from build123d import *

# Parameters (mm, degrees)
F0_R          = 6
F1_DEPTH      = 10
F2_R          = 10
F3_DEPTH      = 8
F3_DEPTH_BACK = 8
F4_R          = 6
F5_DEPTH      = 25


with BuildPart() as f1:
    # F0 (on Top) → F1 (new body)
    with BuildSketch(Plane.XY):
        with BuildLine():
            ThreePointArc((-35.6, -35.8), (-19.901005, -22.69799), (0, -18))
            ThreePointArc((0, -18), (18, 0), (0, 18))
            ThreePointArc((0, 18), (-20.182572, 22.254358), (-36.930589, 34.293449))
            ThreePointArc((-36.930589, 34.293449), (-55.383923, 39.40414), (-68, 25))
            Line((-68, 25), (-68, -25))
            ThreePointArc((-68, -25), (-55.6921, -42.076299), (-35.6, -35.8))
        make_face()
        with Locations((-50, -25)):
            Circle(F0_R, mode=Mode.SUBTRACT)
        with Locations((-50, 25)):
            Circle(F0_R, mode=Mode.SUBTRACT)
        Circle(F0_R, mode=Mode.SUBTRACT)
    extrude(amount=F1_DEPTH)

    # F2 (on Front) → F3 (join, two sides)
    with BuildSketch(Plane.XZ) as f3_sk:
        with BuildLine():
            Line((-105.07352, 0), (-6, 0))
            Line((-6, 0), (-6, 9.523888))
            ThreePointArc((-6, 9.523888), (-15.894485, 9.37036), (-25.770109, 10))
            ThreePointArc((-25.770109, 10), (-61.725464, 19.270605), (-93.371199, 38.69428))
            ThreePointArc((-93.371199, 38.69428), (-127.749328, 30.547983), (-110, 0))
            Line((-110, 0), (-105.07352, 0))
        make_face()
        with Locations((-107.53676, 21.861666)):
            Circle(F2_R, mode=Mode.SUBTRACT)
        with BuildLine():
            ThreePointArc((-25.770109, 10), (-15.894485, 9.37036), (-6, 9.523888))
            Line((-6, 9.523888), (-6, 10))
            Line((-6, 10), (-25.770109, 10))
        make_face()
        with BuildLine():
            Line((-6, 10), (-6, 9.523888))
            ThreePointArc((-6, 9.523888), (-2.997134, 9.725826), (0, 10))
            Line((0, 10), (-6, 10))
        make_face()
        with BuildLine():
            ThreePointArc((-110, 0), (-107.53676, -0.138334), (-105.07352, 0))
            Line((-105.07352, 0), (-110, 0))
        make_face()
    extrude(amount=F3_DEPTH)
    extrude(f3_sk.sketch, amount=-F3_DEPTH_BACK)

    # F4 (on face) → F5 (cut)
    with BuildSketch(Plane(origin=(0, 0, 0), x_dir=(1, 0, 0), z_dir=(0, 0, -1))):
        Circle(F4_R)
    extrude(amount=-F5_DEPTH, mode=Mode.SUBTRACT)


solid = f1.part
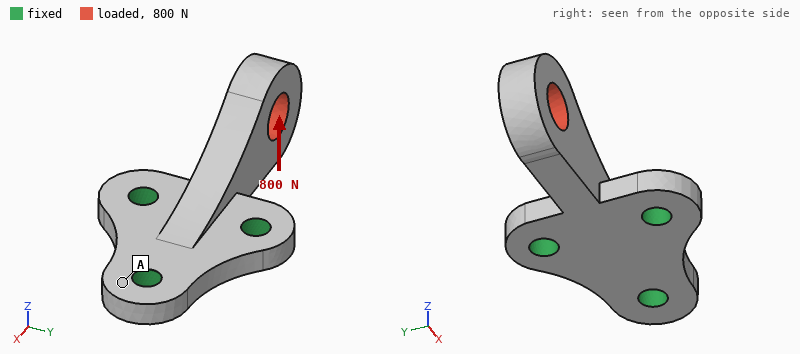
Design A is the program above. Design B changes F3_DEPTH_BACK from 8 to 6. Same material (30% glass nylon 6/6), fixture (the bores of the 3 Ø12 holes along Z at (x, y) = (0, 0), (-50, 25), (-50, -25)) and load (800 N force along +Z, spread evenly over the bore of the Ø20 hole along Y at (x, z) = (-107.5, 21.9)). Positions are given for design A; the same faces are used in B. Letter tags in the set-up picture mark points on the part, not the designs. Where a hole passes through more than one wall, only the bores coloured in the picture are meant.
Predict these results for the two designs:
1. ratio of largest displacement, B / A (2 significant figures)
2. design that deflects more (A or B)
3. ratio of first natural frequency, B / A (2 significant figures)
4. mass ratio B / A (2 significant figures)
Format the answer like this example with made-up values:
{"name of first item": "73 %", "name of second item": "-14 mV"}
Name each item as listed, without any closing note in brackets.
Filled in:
{"ratio of largest displacement, B / A": "1.1", "design that deflects more": "B", "ratio of first natural frequency, B / A": "1.0", "mass ratio B / A": "0.95"}
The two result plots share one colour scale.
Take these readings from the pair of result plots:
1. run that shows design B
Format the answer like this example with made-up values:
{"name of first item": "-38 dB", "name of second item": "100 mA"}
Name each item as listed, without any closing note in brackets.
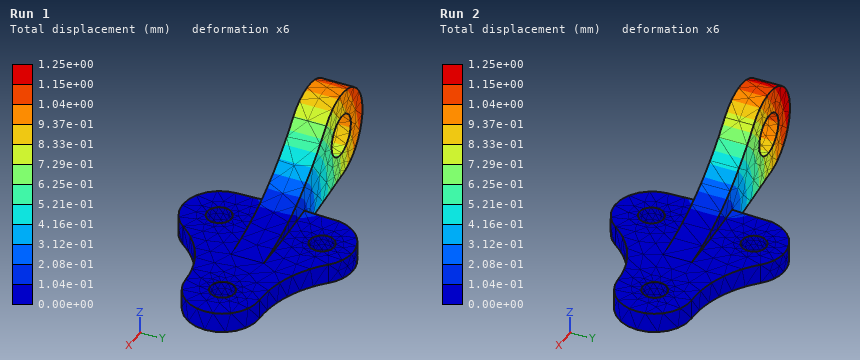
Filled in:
{"run that shows design B": "Run 2"}
